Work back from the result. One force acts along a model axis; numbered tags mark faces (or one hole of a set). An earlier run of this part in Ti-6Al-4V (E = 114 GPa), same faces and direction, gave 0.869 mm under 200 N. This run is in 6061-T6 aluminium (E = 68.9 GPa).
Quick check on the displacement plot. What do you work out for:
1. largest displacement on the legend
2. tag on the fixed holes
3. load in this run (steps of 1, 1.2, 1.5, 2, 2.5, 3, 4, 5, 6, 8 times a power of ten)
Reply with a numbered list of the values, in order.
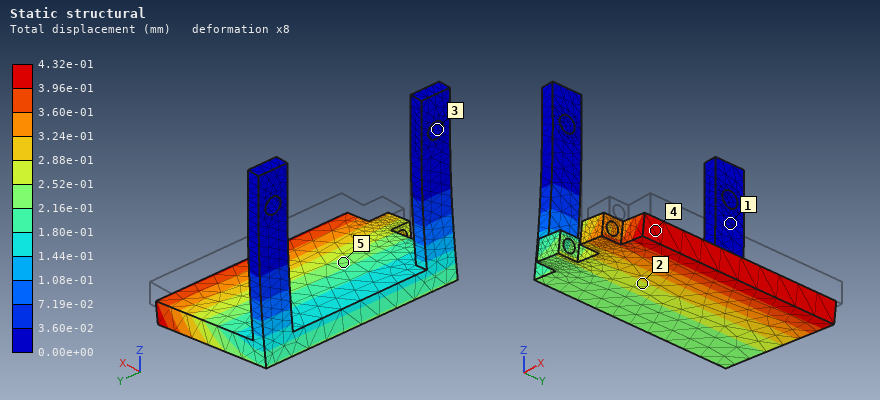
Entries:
1. 4.32e-01 mm
2. 3
3. 60 N
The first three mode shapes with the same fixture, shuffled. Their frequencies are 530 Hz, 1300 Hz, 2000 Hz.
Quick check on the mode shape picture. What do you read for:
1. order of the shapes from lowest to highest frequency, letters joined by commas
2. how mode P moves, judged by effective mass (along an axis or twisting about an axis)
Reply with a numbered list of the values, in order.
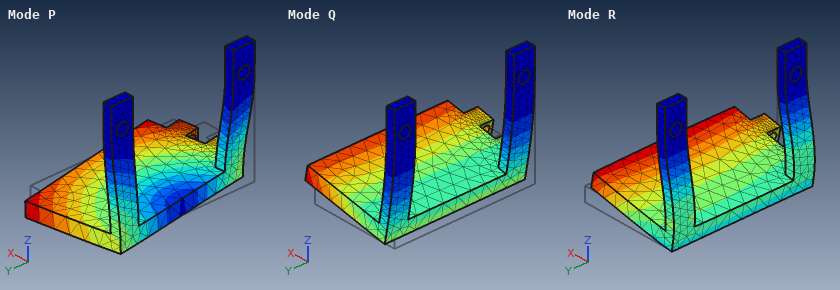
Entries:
1. Q, P, R
2. along Y
